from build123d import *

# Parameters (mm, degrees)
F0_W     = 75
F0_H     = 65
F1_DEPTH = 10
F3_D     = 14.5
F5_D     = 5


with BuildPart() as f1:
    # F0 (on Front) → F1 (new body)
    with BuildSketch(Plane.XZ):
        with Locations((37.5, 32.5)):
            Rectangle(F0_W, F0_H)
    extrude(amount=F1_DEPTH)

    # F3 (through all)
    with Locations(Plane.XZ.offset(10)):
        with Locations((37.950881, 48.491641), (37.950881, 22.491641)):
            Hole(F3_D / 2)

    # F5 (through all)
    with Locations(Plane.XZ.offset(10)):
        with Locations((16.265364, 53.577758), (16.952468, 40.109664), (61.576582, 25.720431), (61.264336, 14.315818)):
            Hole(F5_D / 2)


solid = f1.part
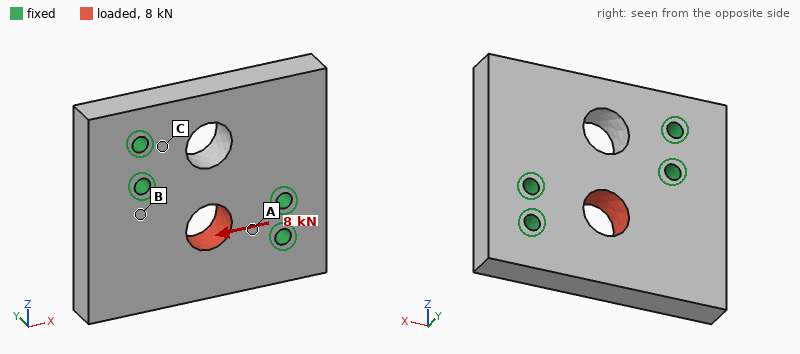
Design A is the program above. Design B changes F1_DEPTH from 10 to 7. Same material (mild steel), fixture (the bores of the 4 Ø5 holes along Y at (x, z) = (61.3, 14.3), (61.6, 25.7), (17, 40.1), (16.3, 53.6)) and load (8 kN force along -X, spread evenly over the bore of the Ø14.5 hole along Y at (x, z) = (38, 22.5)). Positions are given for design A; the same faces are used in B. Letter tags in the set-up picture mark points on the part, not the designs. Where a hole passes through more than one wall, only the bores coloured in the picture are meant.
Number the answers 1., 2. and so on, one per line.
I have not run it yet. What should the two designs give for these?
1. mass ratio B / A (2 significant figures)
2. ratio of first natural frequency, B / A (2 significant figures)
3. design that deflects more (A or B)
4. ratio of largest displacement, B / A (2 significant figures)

1. 0.70
2. 0.75
3. B
4. 1.4
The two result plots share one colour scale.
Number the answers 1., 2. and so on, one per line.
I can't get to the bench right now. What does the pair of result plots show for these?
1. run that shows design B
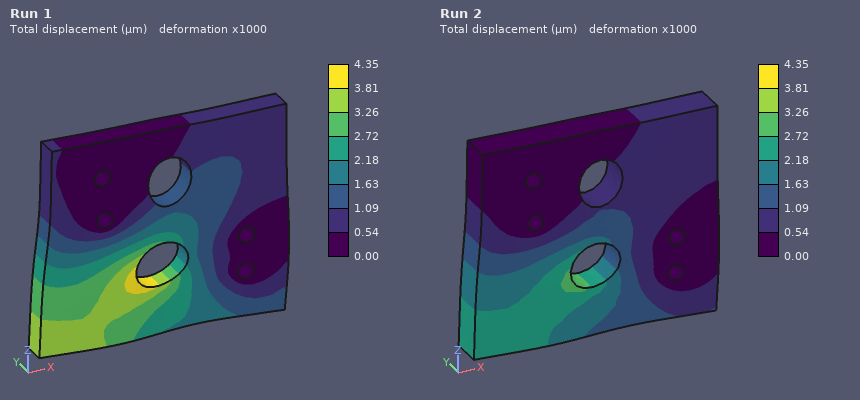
1. Run 1
